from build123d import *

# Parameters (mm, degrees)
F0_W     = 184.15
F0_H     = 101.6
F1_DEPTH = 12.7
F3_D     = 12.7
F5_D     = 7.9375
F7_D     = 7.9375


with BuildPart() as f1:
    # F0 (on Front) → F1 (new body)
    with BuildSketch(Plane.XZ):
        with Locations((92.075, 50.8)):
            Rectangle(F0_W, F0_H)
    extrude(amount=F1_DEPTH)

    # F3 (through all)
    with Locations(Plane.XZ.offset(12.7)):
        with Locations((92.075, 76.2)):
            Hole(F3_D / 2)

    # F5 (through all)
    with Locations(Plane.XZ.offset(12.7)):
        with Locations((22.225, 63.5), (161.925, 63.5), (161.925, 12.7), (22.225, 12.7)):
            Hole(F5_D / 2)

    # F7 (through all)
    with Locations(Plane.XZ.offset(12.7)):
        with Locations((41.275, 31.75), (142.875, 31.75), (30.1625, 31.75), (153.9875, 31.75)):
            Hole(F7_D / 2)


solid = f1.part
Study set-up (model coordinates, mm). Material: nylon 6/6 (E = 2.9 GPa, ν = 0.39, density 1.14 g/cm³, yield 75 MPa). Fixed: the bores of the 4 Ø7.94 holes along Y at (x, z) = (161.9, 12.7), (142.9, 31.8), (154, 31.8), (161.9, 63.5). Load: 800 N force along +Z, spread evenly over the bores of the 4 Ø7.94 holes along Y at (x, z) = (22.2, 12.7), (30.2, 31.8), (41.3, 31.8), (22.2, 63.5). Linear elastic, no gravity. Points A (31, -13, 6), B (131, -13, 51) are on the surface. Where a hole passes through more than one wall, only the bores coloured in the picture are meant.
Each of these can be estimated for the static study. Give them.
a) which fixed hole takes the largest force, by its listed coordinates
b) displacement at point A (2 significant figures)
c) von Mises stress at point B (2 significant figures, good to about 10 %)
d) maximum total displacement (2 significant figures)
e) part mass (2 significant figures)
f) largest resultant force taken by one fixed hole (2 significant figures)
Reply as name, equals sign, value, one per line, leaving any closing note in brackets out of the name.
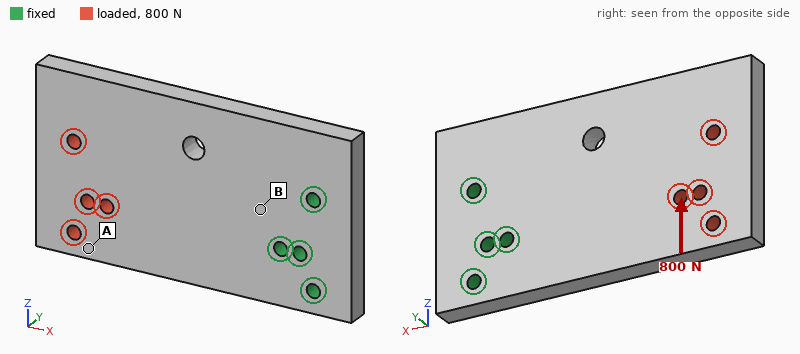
which fixed hole takes the largest force, by its listed coordinates = (161.9, 63.5)
displacement at point A = 0.40 mm
von Mises stress at point B = 3.1 MPa
maximum total displacement = 0.51 mm
part mass = 260 g
largest resultant force taken by one fixed hole = 1.7 kN
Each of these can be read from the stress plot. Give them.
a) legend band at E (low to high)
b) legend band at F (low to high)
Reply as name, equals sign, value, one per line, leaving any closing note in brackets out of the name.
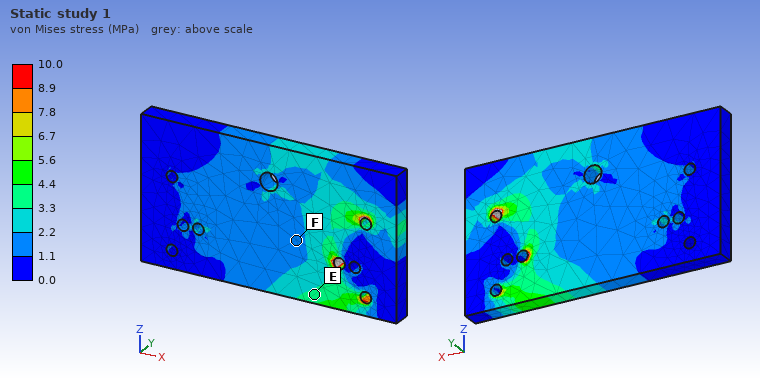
legend band at E = 3.3 to 4.4 MPa
legend band at F = 1.1 to 2.2 MPa
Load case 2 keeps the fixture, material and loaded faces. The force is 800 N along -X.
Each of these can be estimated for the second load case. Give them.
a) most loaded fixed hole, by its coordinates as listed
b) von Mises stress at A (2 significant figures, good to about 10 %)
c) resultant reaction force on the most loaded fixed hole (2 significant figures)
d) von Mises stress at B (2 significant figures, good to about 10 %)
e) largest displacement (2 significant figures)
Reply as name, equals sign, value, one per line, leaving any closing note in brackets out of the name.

most loaded fixed hole, by its coordinates as listed = (142.9, 31.8)
von Mises stress at A = 0.83 MPa
resultant reaction force on the most loaded fixed hole = 310 N
von Mises stress at B = 0.57 MPa
largest displacement = 56 µm
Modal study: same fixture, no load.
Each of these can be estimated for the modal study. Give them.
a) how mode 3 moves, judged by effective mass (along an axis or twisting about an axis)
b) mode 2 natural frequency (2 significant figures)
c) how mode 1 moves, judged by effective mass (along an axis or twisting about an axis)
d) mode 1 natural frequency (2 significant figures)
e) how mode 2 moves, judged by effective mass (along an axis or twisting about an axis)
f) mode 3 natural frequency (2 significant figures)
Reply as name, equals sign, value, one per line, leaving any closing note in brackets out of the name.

how mode 3 moves, judged by effective mass = along Z
mode 2 natural frequency = 410 Hz
how mode 1 moves, judged by effective mass = along Y
mode 1 natural frequency = 150 Hz
how mode 2 moves, judged by effective mass = twisting about X
mode 3 natural frequency = 680 Hz
